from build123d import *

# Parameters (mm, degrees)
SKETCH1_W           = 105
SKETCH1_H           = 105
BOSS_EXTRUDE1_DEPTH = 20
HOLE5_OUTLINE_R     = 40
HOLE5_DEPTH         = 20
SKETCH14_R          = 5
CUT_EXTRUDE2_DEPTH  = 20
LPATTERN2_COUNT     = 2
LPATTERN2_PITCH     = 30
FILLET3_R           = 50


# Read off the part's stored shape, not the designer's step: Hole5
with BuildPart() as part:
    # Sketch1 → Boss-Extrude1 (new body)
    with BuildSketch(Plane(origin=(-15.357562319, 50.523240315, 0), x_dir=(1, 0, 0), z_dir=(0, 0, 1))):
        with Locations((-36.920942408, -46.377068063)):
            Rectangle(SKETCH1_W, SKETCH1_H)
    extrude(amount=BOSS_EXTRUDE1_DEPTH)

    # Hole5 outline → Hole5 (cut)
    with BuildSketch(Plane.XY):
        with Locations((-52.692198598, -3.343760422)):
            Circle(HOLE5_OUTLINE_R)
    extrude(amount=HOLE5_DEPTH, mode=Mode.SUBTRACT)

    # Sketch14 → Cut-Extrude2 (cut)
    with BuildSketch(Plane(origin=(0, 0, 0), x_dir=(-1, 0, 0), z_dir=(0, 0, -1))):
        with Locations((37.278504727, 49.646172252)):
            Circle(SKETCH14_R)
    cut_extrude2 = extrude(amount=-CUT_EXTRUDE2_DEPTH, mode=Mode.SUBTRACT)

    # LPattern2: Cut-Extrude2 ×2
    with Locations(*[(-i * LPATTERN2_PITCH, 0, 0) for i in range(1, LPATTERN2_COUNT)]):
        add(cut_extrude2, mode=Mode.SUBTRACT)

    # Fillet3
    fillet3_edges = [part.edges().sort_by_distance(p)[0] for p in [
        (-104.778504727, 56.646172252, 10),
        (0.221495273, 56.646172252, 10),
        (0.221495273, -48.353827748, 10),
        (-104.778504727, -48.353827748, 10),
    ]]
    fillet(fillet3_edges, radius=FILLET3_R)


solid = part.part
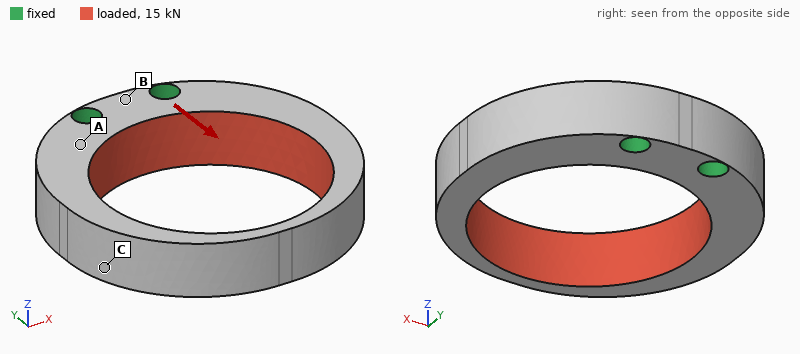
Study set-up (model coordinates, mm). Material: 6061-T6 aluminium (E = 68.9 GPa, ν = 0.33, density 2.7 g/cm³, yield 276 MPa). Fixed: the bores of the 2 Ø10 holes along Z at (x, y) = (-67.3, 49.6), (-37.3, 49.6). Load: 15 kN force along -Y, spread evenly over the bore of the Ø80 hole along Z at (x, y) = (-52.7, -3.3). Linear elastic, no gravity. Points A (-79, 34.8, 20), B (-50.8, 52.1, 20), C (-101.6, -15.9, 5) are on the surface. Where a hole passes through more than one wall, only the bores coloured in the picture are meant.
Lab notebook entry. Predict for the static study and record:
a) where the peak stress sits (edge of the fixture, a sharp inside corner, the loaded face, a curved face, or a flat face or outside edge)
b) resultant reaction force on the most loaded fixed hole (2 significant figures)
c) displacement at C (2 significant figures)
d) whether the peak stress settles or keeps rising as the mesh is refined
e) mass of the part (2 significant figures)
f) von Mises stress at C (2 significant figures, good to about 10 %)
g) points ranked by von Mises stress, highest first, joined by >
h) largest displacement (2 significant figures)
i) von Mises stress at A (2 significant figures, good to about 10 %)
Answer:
edge of the fixture
9.1 kN
0.18 mm
keeps rising
200 g
62 MPa
C > A > B
0.34 mm
37 MPa
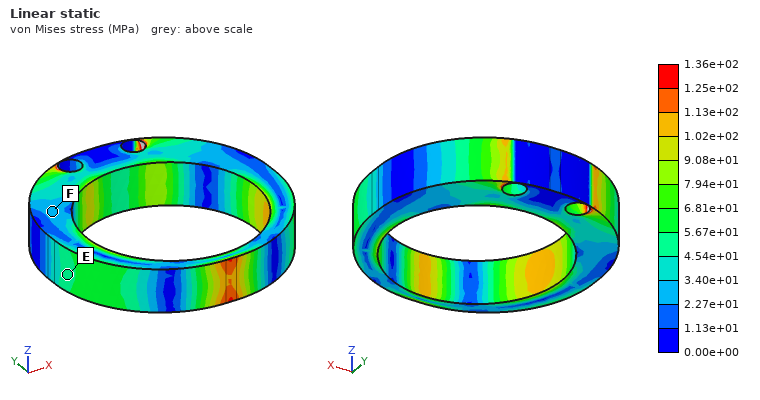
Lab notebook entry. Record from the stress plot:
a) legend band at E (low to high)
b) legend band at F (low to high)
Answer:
4.54e+01 to 5.67e+01 MPa
2.27e+01 to 3.40e+01 MPa
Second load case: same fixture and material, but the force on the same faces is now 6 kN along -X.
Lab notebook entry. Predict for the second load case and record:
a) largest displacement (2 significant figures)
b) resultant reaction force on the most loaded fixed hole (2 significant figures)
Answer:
0.50 mm
5.8 kN
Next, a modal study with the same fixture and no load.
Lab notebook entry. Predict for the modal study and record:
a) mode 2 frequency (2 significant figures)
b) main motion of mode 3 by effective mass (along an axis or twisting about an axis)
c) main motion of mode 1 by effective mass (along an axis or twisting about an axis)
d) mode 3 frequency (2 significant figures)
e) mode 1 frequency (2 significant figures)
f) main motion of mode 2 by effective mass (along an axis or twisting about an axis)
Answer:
1800 Hz
twisting about Y
along Z
2800 Hz
1500 Hz
along X
